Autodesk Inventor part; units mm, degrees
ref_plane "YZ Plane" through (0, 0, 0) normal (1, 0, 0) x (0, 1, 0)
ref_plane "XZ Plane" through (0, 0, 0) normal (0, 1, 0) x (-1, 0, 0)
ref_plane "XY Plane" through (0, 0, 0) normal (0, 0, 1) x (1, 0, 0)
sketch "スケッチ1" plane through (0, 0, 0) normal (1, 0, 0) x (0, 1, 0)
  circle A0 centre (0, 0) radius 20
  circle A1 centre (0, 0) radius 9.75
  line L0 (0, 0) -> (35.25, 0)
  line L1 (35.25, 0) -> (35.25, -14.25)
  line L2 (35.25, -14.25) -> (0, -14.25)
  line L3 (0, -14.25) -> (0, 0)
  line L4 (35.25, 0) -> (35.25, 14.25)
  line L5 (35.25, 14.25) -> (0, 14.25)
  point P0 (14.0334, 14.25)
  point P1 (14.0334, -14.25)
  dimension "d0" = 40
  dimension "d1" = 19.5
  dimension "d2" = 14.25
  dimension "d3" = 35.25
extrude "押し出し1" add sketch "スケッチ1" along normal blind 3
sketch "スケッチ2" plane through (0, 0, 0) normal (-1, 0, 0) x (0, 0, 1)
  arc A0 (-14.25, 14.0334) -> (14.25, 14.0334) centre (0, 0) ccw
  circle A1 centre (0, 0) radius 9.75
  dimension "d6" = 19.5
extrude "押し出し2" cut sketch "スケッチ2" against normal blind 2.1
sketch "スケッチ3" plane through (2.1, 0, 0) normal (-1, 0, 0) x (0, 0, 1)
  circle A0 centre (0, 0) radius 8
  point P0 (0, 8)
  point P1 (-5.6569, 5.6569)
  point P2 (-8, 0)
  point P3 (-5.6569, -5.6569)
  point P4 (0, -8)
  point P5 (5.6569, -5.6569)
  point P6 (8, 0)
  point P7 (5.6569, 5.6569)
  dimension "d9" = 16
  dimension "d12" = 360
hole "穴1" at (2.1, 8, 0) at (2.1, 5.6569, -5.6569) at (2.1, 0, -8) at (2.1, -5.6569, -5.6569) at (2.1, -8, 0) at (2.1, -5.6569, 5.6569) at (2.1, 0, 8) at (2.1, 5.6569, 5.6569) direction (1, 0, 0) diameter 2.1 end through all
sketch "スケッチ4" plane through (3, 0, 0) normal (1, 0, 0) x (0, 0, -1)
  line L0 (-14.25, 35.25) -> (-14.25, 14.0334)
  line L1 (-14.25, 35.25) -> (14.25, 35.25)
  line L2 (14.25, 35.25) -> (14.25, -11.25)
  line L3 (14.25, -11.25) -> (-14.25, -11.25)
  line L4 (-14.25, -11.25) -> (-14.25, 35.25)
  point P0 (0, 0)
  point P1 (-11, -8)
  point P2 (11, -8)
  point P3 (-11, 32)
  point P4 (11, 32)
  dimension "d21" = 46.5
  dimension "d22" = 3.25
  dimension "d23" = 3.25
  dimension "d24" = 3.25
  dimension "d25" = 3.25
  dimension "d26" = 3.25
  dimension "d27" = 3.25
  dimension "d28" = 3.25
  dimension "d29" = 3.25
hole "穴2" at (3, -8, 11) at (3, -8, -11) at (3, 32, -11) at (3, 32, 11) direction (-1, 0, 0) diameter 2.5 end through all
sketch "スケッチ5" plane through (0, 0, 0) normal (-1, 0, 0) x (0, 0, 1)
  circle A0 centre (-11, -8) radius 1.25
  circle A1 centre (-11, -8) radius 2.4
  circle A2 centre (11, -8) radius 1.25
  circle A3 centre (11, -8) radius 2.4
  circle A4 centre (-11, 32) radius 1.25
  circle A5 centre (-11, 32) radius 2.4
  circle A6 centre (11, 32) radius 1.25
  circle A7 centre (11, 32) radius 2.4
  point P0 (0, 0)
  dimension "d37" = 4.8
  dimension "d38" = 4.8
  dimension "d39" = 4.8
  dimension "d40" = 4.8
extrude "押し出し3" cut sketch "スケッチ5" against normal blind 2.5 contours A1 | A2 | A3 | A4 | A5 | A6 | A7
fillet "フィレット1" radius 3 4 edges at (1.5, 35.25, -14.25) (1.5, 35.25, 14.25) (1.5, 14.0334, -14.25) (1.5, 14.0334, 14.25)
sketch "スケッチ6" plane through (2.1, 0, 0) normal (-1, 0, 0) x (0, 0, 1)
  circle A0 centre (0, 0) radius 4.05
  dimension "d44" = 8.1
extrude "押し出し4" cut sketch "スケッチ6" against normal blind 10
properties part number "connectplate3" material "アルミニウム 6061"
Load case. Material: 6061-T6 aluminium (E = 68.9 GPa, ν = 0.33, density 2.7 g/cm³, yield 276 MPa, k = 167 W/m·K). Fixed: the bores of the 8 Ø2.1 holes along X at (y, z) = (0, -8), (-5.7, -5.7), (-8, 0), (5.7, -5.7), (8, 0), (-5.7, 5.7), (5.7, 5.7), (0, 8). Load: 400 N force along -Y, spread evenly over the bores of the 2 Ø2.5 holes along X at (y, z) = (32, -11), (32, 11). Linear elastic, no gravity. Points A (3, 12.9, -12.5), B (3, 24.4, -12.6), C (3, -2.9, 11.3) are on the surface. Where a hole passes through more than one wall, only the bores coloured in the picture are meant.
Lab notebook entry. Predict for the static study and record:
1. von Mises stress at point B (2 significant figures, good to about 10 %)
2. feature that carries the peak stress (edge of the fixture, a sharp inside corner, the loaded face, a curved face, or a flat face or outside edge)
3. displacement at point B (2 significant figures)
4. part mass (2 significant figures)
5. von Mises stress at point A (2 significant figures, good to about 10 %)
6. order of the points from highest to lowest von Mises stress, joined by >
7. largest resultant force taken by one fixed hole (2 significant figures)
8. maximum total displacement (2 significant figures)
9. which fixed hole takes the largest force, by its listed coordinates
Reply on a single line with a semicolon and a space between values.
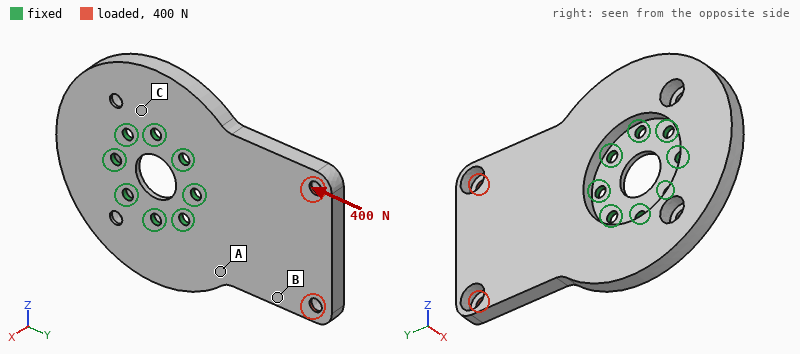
21 MPa; the loaded face; 16 µm; 12 g; 14 MPa; B > A > C; 130 N; 45 µm; (8, 0)
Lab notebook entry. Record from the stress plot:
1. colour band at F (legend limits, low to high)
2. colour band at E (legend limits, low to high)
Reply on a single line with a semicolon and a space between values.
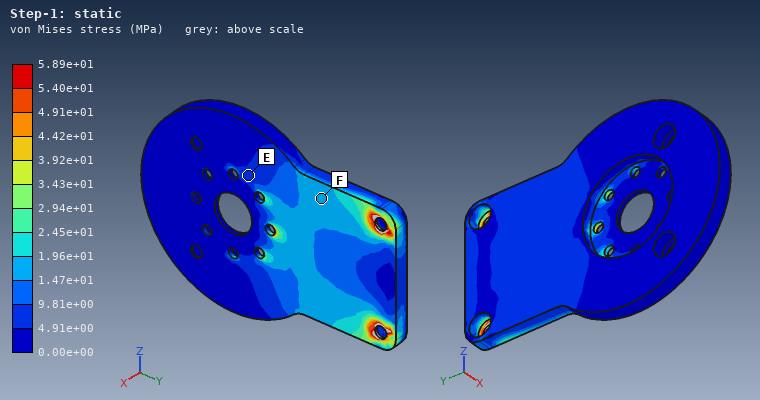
1.47e+01 to 1.96e+01 MPa; 4.91e+00 to 9.81e+00 MPa
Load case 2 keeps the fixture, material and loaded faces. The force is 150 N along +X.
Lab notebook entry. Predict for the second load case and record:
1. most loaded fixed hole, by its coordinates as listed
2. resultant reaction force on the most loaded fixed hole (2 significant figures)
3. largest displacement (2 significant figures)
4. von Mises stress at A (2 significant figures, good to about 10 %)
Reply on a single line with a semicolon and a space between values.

(8, 0); 490 N; 0.36 mm; 66 MPa
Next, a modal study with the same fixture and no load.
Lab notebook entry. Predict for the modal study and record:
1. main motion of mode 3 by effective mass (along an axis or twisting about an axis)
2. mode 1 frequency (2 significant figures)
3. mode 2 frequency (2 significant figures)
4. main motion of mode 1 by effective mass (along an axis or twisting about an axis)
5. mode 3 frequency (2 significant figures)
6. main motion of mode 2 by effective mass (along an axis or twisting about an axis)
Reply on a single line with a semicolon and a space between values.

along X; 2300 Hz; 5300 Hz; along X; 8400 Hz; twisting about Y
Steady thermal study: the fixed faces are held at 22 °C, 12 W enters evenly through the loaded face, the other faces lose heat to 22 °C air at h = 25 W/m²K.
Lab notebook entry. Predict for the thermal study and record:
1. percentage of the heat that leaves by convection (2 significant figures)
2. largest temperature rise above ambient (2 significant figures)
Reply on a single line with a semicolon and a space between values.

7.1 %; 39 K
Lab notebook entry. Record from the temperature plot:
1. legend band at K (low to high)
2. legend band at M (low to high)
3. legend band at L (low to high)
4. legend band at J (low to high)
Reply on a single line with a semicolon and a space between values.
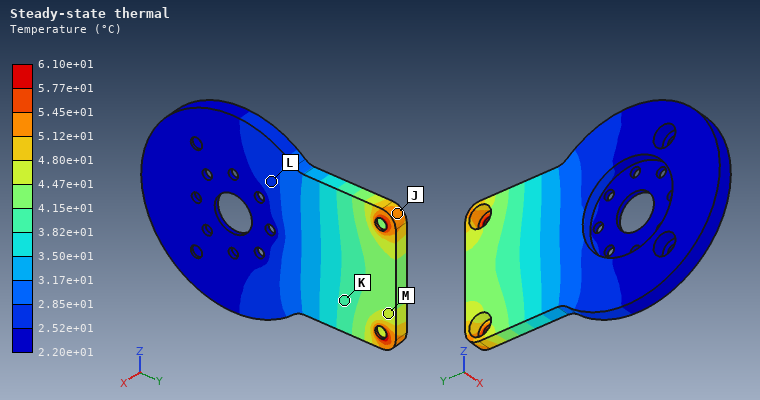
3.82e+01 to 4.15e+01 °C; 4.47e+01 to 4.80e+01 °C; 2.52e+01 to 2.85e+01 °C; 5.12e+01 to 5.45e+01 °C
